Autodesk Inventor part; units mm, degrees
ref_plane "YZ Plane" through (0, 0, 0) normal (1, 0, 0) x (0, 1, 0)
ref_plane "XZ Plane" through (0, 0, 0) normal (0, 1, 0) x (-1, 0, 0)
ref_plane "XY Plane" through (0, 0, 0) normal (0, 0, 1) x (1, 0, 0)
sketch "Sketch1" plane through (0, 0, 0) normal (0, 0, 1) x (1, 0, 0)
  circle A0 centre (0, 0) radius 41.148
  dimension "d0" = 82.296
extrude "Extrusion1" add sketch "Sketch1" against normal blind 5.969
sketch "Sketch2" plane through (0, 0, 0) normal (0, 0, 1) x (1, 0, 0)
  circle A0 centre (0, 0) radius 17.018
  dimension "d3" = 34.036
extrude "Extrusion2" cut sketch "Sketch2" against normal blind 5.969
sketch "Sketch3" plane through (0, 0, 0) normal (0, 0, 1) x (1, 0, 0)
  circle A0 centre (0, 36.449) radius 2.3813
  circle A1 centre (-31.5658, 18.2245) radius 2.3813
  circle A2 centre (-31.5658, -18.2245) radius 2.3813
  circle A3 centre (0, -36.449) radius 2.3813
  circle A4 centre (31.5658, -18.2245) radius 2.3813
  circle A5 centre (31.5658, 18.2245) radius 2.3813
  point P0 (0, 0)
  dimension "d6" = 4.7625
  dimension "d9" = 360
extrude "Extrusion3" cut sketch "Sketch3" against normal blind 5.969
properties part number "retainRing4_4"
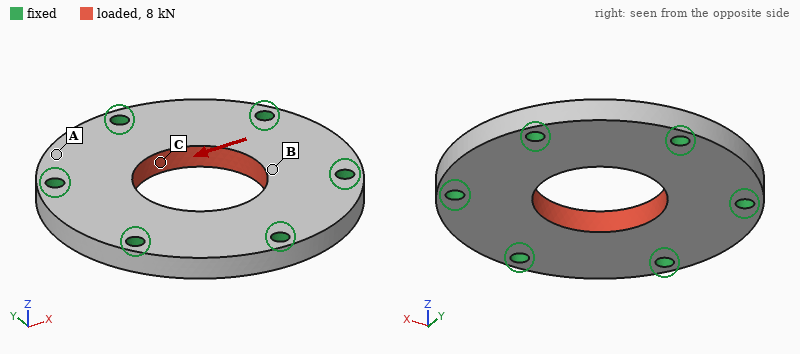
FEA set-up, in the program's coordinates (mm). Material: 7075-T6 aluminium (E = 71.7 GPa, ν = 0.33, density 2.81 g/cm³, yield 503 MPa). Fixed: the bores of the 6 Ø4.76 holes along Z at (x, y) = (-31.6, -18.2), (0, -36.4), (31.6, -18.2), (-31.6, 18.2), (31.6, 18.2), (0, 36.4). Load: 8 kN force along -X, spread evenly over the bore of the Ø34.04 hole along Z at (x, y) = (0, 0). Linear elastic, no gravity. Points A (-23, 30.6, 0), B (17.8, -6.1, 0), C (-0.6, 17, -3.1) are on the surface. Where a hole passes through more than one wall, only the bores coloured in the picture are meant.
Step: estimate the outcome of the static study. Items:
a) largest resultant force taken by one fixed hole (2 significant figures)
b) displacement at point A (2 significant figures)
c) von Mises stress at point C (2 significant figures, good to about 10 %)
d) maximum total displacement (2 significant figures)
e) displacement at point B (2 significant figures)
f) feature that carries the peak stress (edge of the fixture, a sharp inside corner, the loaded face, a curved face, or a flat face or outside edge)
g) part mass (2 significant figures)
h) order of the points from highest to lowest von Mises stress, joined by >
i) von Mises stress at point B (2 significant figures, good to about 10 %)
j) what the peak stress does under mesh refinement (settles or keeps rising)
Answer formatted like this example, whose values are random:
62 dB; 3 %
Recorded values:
1.7 kN; 2.2 µm; 21 MPa; 5.7 µm; 5.0 µm; edge of the fixture; 72 g; C > B > A; 11 MPa; keeps rising
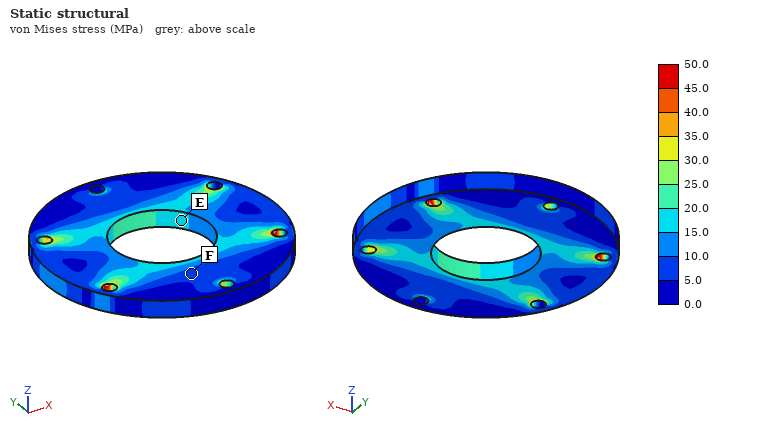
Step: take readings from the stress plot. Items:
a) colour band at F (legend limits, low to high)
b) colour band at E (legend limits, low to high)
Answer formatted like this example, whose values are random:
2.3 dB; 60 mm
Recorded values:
5.0 to 10.0 MPa; 15.0 to 20.0 MPa
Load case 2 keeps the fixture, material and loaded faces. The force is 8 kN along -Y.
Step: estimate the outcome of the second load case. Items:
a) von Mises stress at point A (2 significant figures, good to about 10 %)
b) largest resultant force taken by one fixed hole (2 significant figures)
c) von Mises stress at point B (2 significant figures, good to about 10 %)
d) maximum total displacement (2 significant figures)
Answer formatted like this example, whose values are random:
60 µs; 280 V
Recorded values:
6.6 MPa; 1.9 kN; 17 MPa; 5.7 µm
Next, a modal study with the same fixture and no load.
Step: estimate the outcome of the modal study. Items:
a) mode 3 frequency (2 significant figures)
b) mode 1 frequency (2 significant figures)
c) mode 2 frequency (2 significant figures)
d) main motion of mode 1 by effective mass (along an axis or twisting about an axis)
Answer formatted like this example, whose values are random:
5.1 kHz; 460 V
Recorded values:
16 kHz; 12 kHz; 16 kHz; along Z
